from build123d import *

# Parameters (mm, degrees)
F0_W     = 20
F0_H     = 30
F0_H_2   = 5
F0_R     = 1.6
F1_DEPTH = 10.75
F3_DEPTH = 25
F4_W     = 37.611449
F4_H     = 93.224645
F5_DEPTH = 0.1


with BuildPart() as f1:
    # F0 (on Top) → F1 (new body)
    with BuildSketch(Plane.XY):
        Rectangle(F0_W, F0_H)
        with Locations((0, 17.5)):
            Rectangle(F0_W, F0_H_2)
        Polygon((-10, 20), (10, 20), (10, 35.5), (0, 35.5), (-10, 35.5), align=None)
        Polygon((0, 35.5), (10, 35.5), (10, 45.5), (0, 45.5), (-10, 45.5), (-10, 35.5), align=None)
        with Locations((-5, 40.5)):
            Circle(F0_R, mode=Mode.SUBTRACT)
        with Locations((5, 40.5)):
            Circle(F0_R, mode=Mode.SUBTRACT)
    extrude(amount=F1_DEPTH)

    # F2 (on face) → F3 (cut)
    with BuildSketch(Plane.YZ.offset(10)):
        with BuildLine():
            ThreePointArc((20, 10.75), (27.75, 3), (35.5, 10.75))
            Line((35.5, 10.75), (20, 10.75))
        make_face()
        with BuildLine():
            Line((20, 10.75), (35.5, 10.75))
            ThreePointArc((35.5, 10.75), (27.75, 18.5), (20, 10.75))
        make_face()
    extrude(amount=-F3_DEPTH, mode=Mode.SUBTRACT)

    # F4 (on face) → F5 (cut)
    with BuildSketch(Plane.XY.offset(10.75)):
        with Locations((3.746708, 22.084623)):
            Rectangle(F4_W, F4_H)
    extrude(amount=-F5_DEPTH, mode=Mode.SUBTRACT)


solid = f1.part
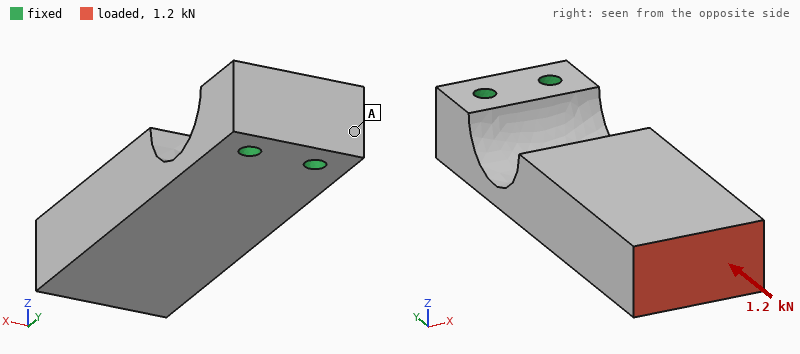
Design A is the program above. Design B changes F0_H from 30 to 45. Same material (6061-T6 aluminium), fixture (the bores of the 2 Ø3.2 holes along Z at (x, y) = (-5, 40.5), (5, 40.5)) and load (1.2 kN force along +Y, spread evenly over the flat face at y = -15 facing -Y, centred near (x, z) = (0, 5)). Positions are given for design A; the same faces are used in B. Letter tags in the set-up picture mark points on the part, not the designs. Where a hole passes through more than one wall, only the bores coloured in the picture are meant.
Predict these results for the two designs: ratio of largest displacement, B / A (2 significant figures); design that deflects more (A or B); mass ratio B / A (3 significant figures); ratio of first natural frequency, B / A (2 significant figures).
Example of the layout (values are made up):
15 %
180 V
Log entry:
1.2
B
1.15
0.79
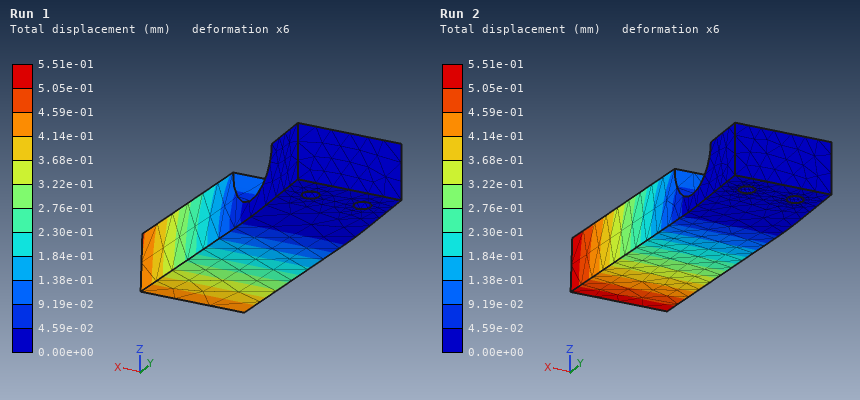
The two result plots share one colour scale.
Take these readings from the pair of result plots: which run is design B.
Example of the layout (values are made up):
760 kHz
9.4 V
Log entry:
Run 2
